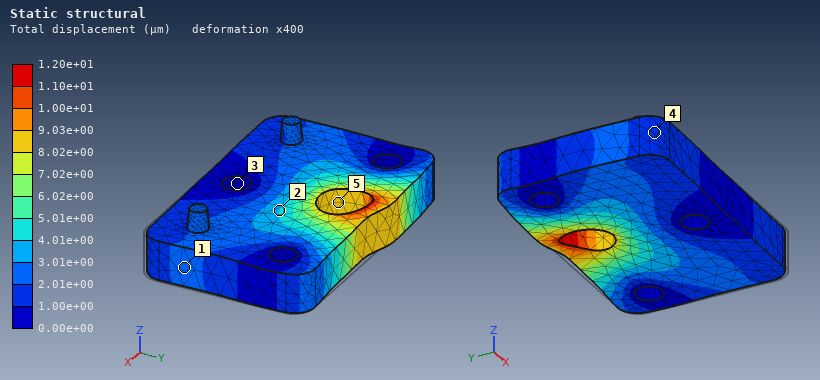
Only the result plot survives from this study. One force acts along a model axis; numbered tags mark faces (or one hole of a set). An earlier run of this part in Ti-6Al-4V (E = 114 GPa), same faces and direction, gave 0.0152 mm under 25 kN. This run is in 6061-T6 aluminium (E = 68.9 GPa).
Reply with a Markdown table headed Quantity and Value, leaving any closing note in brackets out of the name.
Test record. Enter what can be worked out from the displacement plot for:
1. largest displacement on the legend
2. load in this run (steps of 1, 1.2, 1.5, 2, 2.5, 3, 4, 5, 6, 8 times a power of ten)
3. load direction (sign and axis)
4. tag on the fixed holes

| Quantity | Value |
|---|---|
| largest displacement on the legend | 1.20e+01 µm |
| load in this run | 12 kN |
| load direction | -X |
| tag on the fixed holes | 3 |
